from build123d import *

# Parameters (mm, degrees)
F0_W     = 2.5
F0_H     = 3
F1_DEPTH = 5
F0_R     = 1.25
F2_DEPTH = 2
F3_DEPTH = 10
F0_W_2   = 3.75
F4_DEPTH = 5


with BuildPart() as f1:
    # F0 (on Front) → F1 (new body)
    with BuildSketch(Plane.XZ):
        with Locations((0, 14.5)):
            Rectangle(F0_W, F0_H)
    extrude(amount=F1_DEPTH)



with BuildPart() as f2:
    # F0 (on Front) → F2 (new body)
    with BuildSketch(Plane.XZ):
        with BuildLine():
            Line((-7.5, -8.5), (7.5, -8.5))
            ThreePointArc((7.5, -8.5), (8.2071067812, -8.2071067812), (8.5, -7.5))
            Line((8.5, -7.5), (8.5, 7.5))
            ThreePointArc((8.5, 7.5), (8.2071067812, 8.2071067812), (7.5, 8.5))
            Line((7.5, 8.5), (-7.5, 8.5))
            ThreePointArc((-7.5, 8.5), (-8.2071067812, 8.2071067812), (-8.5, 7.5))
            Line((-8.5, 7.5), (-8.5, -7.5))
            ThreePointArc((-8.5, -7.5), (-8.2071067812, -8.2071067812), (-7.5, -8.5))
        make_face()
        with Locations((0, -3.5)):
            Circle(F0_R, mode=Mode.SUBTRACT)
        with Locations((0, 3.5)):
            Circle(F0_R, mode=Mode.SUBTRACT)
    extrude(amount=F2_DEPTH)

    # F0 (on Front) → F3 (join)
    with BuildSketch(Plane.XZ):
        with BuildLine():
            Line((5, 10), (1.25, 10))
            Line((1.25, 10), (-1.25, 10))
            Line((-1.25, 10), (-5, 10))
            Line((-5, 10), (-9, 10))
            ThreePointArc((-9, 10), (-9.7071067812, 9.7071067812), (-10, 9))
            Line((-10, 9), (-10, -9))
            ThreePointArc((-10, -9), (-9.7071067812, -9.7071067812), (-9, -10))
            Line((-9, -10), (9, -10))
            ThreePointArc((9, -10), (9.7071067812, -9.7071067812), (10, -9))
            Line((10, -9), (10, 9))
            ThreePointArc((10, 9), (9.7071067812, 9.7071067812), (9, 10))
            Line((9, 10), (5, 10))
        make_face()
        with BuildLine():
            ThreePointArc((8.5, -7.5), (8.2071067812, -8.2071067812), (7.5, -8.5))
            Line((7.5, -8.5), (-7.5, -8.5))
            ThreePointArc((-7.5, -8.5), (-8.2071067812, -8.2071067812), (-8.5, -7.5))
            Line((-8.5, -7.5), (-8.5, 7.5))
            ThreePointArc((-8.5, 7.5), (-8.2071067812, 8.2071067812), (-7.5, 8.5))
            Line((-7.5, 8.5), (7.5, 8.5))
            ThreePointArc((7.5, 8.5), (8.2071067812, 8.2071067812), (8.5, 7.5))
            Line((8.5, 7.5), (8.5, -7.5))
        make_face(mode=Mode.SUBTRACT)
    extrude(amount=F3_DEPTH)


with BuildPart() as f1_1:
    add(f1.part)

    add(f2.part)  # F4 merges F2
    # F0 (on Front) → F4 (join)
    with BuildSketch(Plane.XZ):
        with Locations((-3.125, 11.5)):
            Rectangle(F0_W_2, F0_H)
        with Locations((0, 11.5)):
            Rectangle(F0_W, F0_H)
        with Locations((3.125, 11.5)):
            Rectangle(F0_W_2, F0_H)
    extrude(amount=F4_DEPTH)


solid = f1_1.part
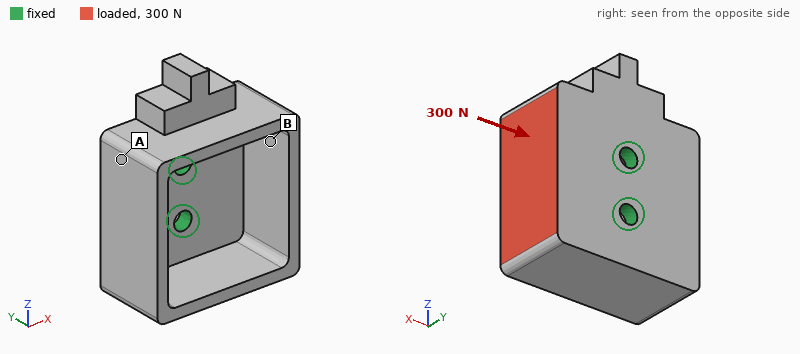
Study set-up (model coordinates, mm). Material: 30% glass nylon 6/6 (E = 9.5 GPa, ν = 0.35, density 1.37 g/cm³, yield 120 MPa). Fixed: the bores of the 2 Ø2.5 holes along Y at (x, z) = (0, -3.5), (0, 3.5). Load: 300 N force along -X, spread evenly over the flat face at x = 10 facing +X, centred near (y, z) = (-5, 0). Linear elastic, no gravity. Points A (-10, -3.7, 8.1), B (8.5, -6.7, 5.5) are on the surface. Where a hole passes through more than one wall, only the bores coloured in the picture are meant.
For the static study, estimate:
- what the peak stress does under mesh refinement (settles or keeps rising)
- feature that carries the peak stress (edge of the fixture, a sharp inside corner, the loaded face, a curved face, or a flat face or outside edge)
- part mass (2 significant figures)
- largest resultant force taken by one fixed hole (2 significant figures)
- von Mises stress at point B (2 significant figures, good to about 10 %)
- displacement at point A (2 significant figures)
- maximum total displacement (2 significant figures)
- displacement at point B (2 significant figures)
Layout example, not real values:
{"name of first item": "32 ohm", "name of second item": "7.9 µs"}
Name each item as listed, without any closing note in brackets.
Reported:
{"what the peak stress does under mesh refinement": "keeps rising", "feature that carries the peak stress": "edge of the fixture", "part mass": "2.5 g", "largest resultant force taken by one fixed hole": "160 N", "von Mises stress at point B": "31 MPa", "displacement at point A": "0.14 mm", "maximum total displacement": "0.37 mm", "displacement at point B": "0.19 mm"}
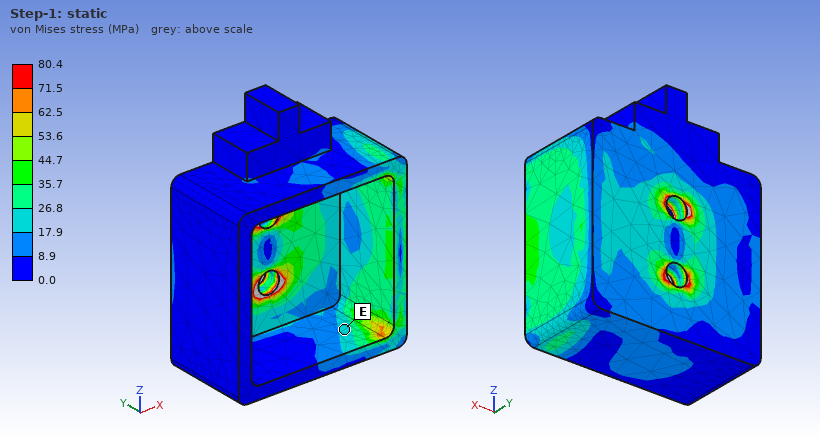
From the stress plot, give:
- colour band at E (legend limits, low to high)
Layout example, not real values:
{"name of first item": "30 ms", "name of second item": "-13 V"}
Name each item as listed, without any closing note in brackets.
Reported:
{"colour band at E": "17.9 to 26.8 MPa"}
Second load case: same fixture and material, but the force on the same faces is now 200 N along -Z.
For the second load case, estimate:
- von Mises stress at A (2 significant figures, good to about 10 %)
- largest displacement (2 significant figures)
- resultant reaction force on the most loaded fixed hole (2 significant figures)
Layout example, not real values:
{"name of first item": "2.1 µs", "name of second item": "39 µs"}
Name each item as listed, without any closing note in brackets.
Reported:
{"von Mises stress at A": "4.6 MPa", "largest displacement": "0.15 mm", "resultant reaction force on the most loaded fixed hole": "250 N"}
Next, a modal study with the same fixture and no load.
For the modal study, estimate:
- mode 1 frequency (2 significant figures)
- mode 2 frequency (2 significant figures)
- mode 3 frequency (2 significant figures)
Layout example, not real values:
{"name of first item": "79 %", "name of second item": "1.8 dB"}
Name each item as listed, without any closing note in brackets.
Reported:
{"mode 1 frequency": "4100 Hz", "mode 2 frequency": "5500 Hz", "mode 3 frequency": "5900 Hz"}
